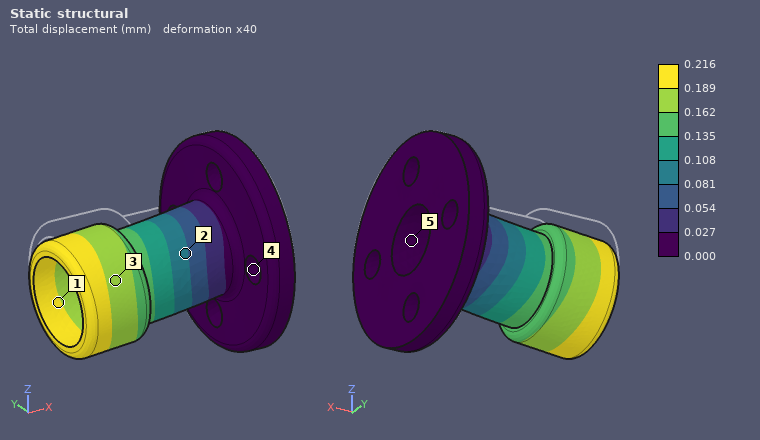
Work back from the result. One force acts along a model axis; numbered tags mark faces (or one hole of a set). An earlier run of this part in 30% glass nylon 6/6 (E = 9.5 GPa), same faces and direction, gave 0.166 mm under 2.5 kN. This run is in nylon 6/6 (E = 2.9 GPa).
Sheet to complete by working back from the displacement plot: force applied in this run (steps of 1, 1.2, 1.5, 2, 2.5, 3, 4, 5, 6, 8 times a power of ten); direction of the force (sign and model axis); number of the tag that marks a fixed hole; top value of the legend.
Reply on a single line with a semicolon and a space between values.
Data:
1 kN; -Z; 4; 0.216 mm
